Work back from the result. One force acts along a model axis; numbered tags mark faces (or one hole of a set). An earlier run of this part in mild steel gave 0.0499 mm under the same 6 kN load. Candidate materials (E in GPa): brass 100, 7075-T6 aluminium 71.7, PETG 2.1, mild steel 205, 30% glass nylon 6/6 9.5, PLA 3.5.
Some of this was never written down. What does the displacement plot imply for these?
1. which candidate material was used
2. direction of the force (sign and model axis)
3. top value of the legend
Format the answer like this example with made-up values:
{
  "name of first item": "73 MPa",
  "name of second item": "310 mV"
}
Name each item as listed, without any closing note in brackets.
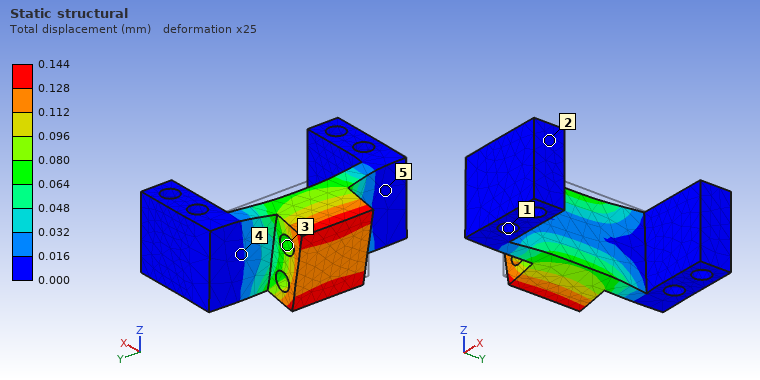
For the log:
{
  "which candidate material was used": "7075-T6 aluminium",
  "direction of the force": "-Z",
  "top value of the legend": "0.144 mm"
}
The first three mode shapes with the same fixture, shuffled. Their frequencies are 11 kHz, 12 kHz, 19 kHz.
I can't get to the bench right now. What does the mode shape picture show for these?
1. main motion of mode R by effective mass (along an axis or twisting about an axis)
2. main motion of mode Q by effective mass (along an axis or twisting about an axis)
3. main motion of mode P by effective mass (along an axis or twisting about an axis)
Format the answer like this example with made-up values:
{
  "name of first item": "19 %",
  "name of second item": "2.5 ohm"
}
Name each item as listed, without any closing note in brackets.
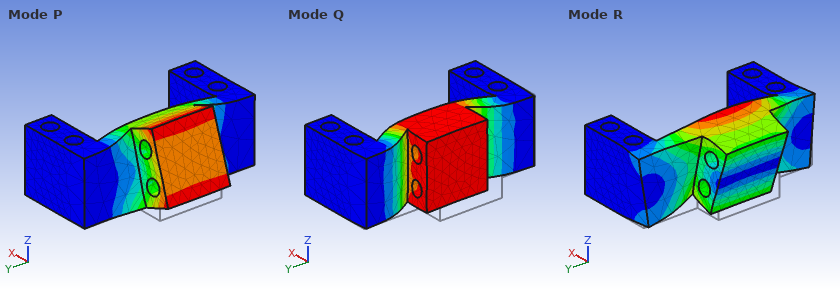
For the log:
{
  "main motion of mode R by effective mass": "along Z",
  "main motion of mode Q by effective mass": "along X",
  "main motion of mode P by effective mass": "along Z"
}
